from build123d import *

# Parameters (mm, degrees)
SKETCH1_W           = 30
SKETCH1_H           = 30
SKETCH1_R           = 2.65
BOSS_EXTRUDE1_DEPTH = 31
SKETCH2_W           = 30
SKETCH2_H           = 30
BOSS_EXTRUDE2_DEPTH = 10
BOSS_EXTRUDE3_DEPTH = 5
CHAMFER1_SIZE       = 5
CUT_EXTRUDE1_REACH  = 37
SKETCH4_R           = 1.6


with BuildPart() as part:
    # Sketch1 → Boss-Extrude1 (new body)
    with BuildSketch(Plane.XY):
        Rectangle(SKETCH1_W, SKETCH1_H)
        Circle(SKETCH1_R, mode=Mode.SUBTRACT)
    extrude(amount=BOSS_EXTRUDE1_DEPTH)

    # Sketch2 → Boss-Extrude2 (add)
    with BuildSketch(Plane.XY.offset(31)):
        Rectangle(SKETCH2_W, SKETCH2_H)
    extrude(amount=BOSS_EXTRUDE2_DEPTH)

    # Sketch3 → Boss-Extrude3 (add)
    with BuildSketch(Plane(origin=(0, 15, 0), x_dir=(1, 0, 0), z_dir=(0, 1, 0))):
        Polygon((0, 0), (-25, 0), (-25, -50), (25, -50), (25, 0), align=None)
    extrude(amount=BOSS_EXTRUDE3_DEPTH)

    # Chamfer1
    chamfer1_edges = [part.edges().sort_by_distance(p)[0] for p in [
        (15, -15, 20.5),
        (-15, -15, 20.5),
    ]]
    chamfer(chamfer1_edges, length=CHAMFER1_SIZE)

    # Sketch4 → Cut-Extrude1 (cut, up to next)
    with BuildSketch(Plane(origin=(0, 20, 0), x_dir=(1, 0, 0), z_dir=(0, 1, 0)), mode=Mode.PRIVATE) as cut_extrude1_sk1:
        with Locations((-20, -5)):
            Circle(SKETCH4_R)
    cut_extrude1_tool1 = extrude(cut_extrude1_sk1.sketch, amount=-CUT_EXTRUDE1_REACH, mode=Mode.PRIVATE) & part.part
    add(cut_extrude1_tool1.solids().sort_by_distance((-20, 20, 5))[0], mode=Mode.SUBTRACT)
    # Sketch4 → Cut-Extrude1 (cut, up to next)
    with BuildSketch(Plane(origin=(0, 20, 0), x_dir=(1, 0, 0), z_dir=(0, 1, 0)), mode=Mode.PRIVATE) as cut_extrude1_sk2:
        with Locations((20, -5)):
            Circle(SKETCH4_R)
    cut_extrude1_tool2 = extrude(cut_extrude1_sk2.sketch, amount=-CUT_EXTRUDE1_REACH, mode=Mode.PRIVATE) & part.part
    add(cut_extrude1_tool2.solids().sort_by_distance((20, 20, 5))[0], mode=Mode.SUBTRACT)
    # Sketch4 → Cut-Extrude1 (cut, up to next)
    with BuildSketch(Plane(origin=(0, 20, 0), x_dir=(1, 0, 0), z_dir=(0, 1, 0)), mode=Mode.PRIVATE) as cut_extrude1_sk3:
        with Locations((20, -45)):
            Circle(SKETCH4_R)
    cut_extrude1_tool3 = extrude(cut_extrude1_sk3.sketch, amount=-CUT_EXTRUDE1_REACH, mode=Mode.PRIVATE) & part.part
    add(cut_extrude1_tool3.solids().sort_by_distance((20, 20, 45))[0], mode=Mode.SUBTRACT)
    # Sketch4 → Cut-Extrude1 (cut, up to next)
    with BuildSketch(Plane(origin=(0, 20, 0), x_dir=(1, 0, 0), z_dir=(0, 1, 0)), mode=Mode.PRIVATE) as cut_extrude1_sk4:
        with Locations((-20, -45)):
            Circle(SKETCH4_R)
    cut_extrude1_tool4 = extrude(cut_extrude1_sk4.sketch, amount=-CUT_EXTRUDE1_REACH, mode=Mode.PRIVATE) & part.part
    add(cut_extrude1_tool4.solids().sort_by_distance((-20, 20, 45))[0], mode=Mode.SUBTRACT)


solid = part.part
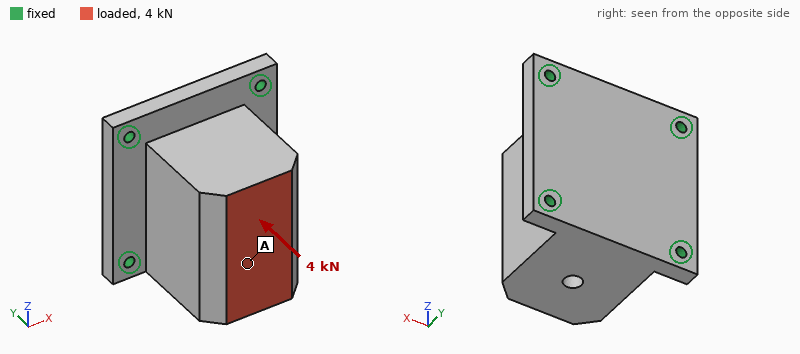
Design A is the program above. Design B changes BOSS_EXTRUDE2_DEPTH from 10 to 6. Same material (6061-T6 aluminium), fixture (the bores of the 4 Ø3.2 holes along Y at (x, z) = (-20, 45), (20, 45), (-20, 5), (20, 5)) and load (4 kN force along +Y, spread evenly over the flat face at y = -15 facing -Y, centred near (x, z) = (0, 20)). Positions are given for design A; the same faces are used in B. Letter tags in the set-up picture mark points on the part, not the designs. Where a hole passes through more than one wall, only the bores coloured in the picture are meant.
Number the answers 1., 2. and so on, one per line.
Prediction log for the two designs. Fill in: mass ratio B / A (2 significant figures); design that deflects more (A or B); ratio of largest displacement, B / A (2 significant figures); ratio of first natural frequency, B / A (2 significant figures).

1. 0.93
2. B
3. 1.4
4. 0.89
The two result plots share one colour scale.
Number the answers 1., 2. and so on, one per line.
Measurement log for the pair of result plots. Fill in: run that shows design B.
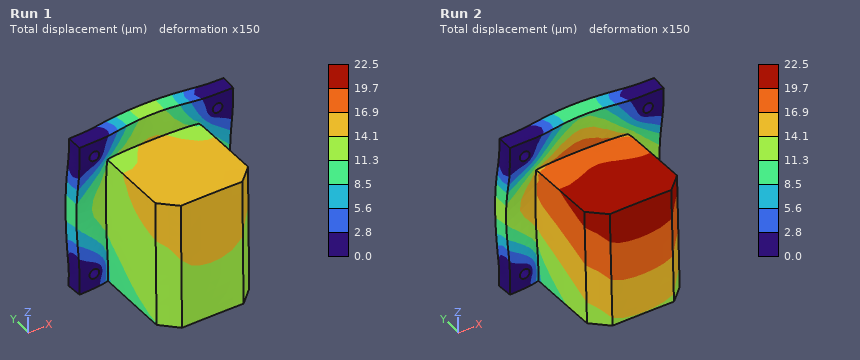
1. Run 2
